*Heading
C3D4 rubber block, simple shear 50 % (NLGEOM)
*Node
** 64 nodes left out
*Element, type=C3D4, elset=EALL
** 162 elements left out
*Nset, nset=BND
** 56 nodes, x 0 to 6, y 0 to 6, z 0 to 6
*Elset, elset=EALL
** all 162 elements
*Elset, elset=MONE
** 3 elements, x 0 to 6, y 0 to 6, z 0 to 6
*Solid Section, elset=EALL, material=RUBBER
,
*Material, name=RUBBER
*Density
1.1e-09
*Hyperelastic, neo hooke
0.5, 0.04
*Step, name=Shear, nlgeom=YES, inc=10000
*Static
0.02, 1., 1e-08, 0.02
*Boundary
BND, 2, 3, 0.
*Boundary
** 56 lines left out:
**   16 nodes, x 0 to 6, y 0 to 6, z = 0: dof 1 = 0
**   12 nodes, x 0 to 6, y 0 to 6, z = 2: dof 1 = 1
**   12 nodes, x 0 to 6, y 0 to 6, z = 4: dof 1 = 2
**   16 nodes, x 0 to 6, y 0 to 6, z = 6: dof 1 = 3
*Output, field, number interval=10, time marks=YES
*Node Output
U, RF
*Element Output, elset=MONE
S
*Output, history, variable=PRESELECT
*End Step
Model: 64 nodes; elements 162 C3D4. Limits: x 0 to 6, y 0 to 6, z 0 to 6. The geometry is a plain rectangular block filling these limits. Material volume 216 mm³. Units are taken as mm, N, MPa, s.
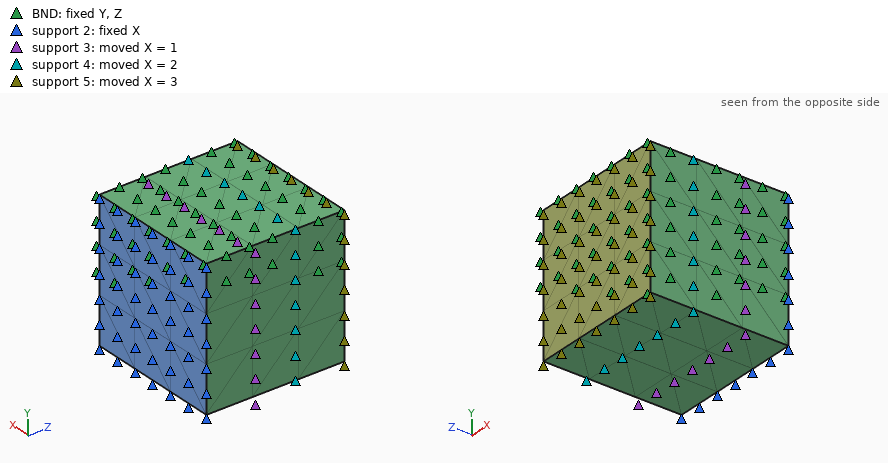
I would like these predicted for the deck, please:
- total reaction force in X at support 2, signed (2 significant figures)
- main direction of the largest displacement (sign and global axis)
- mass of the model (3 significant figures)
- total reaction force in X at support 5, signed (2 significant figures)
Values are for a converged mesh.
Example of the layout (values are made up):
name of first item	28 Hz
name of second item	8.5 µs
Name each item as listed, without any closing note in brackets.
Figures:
total reaction force in X at support 2, signed	-18 N
main direction of the largest displacement	+X
mass of the model	2.38e-04 kg
total reaction force in X at support 5, signed	18 N
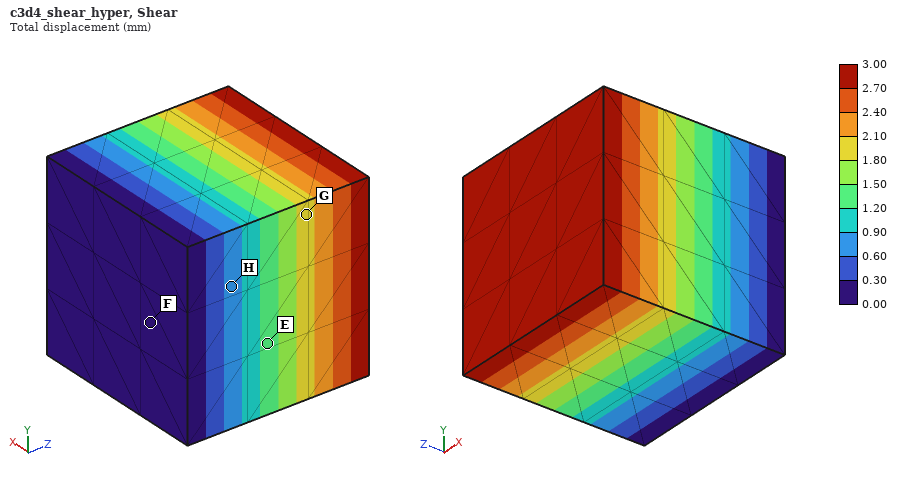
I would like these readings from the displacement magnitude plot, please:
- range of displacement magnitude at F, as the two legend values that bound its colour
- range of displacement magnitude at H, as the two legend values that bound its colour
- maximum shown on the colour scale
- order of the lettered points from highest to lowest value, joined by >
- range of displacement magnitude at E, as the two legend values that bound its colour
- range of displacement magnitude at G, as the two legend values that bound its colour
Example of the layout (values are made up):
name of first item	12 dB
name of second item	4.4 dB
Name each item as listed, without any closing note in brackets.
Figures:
range of displacement magnitude at F, as the two legend values that bound its colour	0.00 to 0.30 mm
range of displacement magnitude at H, as the two legend values that bound its colour	0.60 to 0.90 mm
maximum shown on the colour scale	3.00 mm
order of the lettered points from highest to lowest value, joined by >	G > E > H > F
range of displacement magnitude at E, as the two legend values that bound its colour	1.20 to 1.50 mm
range of displacement magnitude at G, as the two legend values that bound its colour	1.80 to 2.10 mm
